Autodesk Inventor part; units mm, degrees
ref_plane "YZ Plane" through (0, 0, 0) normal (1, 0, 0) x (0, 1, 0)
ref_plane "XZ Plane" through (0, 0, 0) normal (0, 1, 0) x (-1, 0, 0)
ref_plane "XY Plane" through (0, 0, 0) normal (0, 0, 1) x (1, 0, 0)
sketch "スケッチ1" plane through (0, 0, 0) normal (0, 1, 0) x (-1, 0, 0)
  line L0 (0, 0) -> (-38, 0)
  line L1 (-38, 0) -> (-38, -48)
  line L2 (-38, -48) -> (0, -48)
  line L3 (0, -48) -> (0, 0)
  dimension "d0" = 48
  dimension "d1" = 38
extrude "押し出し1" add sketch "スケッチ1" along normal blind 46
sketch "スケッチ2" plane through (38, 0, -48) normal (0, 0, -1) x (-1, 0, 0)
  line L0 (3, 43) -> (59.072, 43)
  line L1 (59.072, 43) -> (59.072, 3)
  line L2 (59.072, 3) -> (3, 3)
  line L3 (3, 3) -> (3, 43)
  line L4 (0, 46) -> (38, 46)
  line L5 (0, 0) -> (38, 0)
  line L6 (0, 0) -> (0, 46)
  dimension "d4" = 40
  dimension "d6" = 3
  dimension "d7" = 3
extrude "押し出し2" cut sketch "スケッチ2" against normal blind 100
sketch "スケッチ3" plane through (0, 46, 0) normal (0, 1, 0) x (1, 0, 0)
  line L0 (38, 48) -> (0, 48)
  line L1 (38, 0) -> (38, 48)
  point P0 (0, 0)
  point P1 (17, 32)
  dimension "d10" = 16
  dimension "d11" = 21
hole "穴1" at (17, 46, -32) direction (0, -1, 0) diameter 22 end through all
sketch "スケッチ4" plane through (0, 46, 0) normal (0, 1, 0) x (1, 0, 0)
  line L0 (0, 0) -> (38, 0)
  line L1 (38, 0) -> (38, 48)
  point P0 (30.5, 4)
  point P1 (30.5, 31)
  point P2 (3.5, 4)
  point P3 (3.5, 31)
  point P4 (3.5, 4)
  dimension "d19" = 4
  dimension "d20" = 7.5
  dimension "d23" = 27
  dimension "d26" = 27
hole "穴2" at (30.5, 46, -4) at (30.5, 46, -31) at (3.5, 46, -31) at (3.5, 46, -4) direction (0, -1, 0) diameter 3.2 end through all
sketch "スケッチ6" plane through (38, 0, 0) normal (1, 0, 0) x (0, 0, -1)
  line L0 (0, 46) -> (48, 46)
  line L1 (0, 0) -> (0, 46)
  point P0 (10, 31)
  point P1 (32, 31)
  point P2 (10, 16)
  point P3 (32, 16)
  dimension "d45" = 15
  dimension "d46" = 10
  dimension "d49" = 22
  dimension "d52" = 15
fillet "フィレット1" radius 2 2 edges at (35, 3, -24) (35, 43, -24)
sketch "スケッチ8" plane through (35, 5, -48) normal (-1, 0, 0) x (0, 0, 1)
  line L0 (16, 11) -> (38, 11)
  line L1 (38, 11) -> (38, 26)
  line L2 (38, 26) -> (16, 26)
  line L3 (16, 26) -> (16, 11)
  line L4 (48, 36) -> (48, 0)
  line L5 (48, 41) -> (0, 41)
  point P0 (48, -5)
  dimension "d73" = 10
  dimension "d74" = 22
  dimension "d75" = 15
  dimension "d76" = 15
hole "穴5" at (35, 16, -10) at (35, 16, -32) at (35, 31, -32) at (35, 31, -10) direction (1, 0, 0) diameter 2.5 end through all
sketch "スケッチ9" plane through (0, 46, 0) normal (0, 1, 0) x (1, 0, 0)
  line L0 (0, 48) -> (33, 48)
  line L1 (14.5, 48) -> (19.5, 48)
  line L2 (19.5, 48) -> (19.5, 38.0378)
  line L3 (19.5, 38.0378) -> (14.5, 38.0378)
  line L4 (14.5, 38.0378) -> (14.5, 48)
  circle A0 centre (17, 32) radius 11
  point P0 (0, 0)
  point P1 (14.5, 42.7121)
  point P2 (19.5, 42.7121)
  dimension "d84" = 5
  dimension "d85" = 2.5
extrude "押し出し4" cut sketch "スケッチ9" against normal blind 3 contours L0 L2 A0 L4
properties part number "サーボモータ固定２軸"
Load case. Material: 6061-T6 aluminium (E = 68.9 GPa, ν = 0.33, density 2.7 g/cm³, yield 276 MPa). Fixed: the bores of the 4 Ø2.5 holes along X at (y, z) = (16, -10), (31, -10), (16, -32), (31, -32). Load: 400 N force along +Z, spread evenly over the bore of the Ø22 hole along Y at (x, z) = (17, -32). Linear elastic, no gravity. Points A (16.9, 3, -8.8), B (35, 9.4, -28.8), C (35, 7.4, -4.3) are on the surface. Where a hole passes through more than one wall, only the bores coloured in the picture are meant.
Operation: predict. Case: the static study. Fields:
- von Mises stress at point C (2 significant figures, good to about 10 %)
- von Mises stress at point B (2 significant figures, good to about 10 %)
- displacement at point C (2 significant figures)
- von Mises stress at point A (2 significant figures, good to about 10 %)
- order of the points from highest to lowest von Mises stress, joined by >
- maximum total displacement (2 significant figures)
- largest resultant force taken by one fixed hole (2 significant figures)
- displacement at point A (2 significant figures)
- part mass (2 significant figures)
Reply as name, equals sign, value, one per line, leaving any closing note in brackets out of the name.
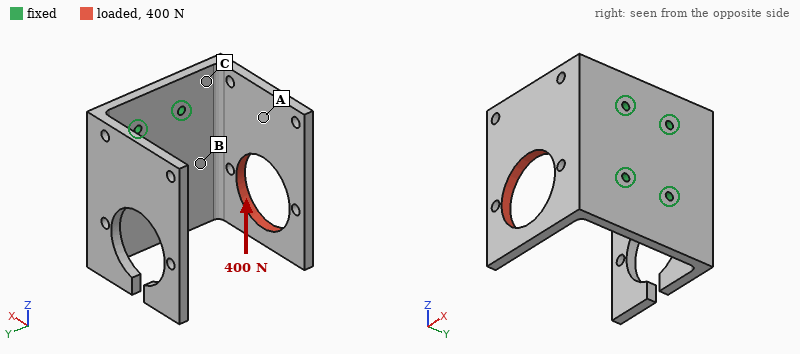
von Mises stress at point C = 28 MPa
von Mises stress at point B = 44 MPa
displacement at point C = 0.037 mm
von Mises stress at point A = 12 MPa
order of the points from highest to lowest von Mises stress, joined by > = B > C > A
maximum total displacement = 0.18 mm
largest resultant force taken by one fixed hole = 440 N
displacement at point A = 0.098 mm
part mass = 38 g
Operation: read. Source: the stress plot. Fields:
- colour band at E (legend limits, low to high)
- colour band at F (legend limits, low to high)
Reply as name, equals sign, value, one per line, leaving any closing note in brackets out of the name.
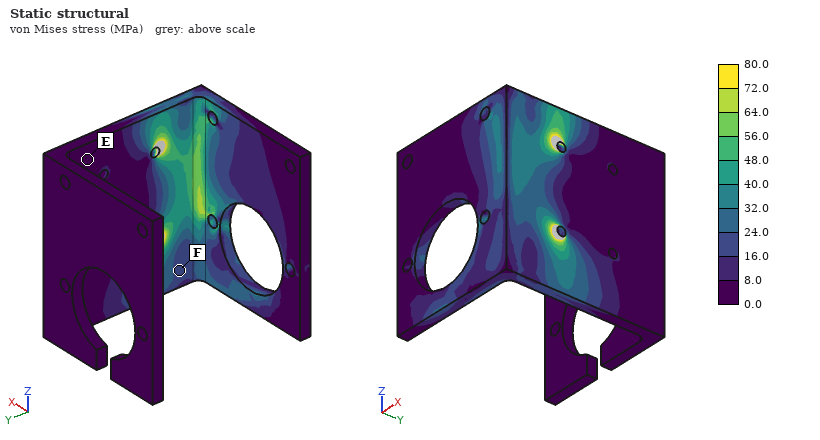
colour band at E = 0.0 to 8.0 MPa
colour band at F = 16.0 to 24.0 MPa
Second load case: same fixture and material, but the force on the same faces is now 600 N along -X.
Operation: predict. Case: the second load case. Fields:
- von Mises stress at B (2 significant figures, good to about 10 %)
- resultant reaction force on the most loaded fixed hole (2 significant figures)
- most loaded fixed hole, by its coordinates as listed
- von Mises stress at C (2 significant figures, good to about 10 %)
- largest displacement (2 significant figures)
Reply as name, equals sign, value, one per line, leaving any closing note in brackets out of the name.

von Mises stress at B = 83 MPa
resultant reaction force on the most loaded fixed hole = 720 N
most loaded fixed hole, by its coordinates as listed = (16, -32)
von Mises stress at C = 49 MPa
largest displacement = 0.44 mm
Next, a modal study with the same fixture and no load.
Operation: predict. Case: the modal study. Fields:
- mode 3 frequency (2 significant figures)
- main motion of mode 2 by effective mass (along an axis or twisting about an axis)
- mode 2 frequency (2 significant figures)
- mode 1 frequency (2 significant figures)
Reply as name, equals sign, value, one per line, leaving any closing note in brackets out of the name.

mode 3 frequency = 1800 Hz
main motion of mode 2 by effective mass = along Y
mode 2 frequency = 1200 Hz
mode 1 frequency = 1000 Hz
